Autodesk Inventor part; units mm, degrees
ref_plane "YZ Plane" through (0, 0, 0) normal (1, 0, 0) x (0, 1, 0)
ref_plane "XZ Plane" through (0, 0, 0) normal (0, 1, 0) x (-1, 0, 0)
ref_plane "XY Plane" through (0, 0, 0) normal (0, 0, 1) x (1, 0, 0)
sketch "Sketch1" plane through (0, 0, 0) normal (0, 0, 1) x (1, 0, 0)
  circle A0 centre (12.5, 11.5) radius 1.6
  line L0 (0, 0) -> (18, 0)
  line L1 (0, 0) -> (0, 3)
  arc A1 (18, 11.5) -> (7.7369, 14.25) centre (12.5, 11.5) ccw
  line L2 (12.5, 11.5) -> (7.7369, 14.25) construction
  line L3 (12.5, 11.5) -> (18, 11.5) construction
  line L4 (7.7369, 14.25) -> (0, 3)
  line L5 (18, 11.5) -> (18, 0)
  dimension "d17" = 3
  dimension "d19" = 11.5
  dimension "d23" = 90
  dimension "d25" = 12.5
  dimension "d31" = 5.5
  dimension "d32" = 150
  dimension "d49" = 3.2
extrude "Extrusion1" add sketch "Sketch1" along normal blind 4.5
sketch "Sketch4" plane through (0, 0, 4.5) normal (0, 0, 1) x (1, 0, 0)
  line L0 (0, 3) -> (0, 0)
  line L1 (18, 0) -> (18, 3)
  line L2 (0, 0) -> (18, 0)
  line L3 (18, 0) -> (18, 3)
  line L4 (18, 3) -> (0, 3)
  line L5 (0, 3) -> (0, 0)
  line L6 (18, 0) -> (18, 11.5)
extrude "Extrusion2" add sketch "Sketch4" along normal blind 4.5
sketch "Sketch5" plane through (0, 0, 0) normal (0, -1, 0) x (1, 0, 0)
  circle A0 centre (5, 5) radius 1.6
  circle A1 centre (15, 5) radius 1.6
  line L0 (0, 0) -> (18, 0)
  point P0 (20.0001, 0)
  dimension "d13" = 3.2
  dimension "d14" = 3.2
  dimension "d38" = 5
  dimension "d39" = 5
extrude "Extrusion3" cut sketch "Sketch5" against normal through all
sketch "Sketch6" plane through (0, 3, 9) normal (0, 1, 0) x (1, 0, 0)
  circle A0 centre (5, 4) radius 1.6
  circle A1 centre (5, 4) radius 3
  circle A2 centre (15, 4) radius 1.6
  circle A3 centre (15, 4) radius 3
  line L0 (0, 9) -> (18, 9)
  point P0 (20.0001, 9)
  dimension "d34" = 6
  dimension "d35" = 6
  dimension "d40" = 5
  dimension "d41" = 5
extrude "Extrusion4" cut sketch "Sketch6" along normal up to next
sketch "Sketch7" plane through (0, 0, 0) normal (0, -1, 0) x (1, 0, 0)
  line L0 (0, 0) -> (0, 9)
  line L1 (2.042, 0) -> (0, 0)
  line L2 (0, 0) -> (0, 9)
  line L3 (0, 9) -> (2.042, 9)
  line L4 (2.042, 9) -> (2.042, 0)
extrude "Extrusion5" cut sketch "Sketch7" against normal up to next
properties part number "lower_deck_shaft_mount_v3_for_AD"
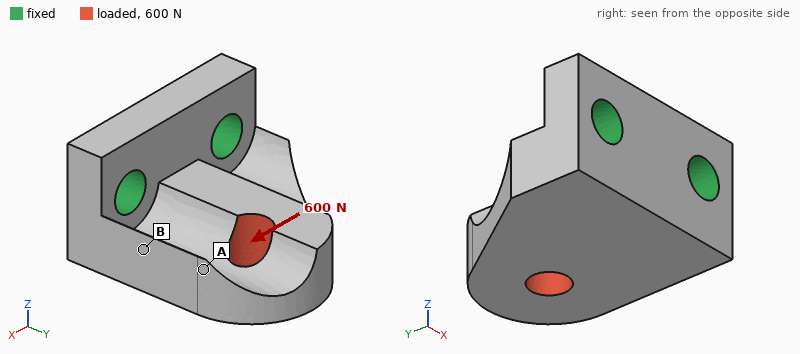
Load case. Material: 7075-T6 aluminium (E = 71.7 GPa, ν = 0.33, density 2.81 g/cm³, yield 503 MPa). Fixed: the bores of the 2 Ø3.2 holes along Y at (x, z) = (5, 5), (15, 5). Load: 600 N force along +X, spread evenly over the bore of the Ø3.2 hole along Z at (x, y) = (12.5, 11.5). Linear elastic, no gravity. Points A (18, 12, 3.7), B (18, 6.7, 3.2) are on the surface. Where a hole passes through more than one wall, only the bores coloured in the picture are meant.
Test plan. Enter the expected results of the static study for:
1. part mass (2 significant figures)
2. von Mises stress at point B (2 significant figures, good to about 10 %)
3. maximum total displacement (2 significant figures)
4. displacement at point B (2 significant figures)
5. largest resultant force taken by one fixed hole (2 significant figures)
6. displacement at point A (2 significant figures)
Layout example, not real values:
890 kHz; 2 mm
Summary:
2.6 g; 40 MPa; 27 µm; 13 µm; 630 N; 23 µm
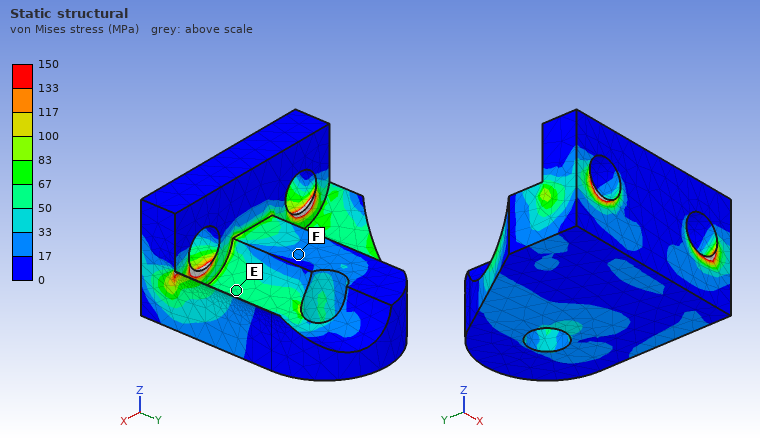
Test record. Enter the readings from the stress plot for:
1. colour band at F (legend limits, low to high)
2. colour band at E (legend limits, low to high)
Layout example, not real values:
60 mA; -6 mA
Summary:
17 to 33 MPa; 50 to 67 MPa
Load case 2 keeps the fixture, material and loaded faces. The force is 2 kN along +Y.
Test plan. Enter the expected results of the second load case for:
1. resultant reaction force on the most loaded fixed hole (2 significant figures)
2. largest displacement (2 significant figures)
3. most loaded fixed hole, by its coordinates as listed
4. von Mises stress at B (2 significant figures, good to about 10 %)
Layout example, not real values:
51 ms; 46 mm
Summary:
1.4 kN; 52 µm; (15, 5); 75 MPa
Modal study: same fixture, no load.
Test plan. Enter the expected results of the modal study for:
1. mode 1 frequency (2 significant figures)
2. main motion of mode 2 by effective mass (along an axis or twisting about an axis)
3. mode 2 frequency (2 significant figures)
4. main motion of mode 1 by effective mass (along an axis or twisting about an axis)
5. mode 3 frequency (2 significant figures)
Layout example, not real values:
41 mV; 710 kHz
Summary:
13 kHz; along X; 27 kHz; along Z; 36 kHz
